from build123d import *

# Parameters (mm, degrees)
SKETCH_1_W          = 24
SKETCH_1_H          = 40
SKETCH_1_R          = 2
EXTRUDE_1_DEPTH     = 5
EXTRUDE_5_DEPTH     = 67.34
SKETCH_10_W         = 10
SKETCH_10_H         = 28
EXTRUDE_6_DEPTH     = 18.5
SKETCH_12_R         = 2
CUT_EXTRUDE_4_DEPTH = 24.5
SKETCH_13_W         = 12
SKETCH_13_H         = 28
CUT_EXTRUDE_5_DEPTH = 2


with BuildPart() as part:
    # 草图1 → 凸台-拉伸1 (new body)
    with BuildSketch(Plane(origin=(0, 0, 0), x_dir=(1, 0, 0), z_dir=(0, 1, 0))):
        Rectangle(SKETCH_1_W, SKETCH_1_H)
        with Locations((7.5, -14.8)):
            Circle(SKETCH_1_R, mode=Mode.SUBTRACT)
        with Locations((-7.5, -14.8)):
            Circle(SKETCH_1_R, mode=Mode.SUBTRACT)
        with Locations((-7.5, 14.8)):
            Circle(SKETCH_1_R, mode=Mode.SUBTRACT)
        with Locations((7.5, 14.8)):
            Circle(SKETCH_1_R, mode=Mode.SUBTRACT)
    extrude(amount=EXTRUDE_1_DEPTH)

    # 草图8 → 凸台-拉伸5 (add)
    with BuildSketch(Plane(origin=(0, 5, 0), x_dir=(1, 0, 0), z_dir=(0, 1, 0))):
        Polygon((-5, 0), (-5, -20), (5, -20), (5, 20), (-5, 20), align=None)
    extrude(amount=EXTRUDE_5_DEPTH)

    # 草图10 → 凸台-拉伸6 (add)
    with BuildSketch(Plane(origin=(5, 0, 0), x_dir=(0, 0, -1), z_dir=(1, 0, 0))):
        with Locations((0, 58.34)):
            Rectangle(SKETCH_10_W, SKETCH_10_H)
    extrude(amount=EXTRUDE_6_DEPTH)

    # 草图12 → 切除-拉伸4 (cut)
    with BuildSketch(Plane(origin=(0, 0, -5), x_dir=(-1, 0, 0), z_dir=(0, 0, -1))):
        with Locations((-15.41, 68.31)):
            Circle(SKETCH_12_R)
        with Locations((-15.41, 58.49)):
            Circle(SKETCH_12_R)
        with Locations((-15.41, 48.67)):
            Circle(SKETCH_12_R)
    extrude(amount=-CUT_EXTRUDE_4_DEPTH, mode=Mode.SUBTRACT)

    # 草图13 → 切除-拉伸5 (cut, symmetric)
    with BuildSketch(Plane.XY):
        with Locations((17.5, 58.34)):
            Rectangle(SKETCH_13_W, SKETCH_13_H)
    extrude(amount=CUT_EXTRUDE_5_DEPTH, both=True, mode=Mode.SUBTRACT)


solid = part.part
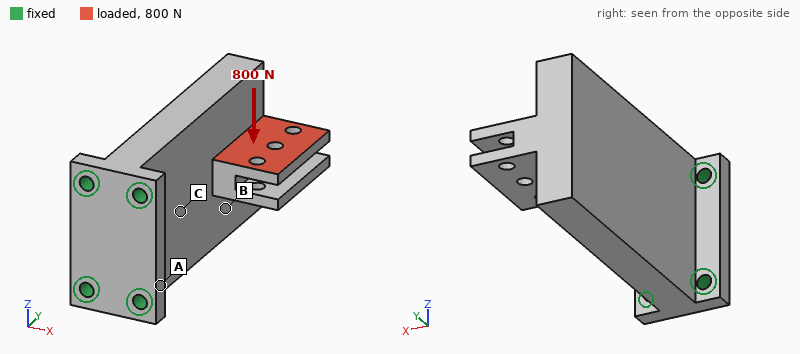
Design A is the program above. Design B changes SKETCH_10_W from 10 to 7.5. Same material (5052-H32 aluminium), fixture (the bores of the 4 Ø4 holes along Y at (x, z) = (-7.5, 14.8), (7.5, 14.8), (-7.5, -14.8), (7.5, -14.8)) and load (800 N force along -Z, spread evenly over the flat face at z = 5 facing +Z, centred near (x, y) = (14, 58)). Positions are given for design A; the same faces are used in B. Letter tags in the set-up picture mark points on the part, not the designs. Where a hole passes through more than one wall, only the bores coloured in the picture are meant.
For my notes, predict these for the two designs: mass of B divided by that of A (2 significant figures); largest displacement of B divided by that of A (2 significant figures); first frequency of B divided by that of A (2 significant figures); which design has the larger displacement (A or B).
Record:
0.97
2.3
1.0
B
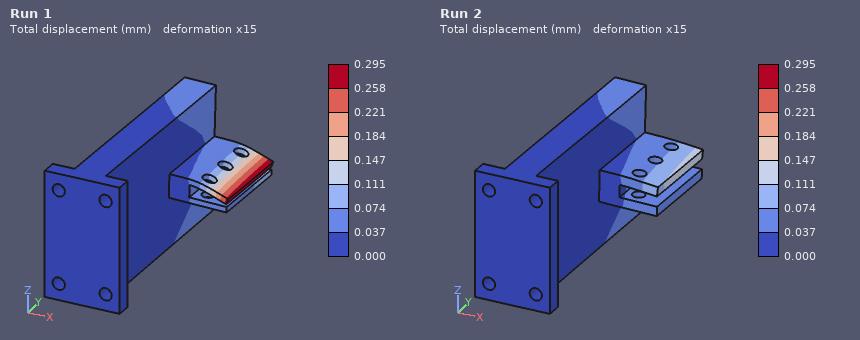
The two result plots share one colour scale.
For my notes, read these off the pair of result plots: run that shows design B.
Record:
Run 1
